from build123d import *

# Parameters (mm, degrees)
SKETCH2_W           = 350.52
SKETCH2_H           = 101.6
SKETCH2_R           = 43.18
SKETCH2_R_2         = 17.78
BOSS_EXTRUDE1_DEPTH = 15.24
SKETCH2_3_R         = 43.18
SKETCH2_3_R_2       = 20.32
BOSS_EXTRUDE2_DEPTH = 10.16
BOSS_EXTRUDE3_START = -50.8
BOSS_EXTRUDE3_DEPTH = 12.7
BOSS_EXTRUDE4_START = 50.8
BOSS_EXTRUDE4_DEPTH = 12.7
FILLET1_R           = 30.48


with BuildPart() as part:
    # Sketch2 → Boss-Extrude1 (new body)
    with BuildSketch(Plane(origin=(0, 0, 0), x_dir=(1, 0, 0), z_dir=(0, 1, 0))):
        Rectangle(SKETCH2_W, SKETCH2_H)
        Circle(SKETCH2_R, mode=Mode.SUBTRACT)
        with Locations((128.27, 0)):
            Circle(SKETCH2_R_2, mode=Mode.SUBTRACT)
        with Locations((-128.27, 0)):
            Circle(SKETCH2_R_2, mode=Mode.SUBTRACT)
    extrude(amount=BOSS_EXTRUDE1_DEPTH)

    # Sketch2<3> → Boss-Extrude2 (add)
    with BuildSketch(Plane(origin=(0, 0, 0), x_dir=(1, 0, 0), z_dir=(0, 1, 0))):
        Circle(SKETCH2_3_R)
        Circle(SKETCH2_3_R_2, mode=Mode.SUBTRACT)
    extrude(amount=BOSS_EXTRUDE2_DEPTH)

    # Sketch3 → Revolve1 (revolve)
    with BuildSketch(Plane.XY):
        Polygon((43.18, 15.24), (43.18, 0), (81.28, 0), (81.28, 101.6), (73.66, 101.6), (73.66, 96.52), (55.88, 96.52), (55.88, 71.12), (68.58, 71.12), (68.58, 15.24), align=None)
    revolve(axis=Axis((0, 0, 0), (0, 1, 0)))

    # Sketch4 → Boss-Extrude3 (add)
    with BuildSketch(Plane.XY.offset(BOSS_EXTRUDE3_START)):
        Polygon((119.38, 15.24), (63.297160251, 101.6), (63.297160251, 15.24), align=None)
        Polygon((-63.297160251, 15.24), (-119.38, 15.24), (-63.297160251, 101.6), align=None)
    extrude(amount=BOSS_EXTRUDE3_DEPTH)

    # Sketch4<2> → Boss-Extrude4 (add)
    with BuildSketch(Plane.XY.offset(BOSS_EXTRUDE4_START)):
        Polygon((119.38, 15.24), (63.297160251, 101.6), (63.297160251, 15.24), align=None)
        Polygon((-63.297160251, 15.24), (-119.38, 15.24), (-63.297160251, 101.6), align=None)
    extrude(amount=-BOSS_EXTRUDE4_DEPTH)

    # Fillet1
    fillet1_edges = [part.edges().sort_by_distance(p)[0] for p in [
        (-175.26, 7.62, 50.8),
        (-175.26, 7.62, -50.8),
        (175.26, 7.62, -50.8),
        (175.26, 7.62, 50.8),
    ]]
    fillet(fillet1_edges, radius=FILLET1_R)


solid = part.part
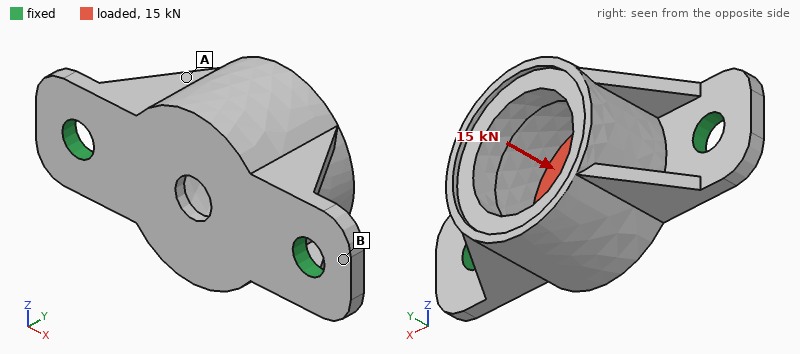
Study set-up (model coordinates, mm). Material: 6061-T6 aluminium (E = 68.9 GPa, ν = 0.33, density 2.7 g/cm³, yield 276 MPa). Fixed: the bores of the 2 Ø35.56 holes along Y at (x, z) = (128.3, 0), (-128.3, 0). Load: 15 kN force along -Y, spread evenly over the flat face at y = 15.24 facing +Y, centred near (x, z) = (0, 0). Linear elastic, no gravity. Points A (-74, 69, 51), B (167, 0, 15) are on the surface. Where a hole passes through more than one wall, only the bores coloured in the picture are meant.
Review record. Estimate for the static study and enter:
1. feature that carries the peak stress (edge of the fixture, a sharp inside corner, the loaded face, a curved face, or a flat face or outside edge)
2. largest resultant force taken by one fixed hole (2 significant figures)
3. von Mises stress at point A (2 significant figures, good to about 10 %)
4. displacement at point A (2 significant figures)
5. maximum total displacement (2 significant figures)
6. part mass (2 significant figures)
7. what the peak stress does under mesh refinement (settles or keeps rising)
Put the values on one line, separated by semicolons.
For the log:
edge of the fixture; 8.4 kN; 10 MPa; 35 µm; 67 µm; 3.4 kg; keeps rising
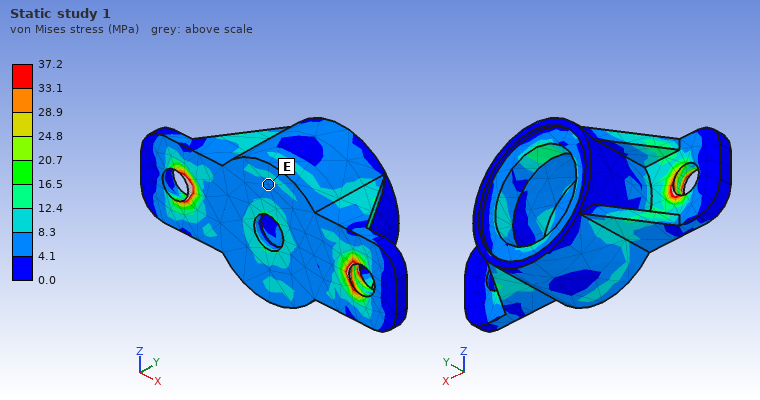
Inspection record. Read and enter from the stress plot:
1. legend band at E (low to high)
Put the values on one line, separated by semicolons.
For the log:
4.1 to 8.3 MPa
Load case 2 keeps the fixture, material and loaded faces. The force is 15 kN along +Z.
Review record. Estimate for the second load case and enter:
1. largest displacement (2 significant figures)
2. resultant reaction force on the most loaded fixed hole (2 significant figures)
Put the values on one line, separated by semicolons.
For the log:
54 µm; 7.5 kN
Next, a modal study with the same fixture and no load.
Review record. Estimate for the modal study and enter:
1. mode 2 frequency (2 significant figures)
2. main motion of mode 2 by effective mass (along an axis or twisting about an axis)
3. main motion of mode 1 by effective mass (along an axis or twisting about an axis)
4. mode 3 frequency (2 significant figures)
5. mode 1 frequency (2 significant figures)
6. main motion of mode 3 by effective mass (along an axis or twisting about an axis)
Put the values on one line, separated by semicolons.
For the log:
1800 Hz; along Y; along Z; 3100 Hz; 910 Hz; along X
